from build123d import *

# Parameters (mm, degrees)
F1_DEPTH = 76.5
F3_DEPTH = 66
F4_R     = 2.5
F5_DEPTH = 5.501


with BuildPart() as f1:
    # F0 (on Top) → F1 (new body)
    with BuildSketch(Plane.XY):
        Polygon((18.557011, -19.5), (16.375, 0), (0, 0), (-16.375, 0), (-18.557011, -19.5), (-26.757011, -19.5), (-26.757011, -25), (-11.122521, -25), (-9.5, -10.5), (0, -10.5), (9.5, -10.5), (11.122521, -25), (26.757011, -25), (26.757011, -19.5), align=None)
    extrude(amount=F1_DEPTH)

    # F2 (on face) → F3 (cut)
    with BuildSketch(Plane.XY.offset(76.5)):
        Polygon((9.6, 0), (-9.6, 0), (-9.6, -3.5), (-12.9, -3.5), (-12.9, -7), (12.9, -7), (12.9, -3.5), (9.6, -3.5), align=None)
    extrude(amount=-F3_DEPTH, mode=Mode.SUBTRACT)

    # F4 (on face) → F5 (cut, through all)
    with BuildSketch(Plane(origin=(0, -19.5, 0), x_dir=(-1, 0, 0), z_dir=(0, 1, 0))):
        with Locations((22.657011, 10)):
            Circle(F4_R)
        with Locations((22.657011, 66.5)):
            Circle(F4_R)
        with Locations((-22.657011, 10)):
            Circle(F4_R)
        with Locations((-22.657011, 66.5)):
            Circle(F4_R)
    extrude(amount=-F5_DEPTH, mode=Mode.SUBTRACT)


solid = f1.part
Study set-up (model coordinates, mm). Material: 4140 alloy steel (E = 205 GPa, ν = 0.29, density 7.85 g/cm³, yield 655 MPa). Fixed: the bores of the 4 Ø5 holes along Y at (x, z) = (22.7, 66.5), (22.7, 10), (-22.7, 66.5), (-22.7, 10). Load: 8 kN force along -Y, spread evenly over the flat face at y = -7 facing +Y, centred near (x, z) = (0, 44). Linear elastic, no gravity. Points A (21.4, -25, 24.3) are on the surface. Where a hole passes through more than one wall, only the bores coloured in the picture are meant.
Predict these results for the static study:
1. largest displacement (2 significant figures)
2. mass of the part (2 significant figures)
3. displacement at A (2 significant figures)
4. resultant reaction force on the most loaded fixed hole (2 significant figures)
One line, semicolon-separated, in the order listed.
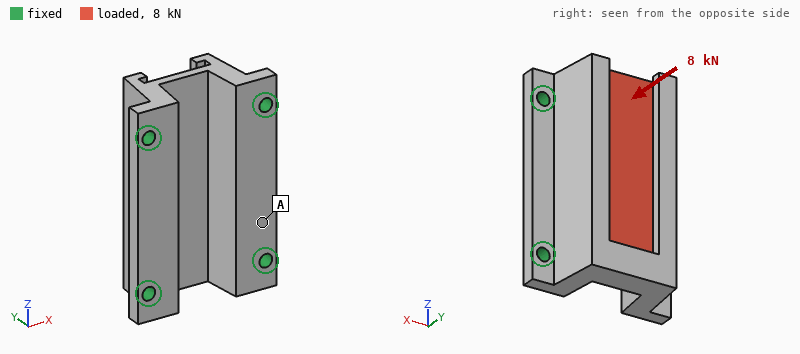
12 µm; 320 g; 4.0 µm; 3.1 kN
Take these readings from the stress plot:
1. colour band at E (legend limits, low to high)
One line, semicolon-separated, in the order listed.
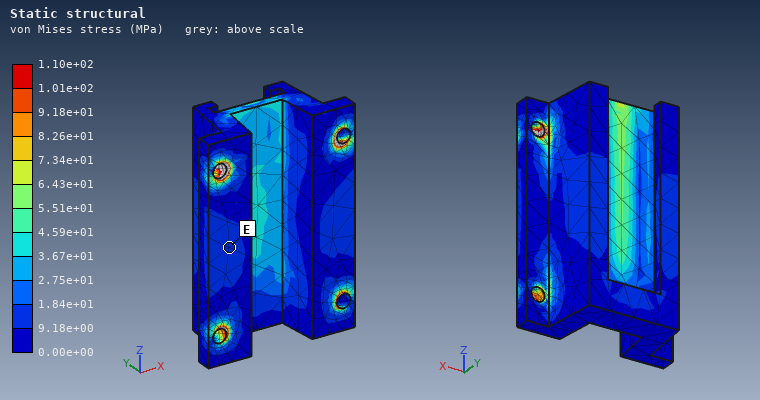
9.18e+00 to 1.84e+01 MPa
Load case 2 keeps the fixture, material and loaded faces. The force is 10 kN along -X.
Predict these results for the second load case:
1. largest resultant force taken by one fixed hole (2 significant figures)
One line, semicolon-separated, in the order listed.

3.2 kN
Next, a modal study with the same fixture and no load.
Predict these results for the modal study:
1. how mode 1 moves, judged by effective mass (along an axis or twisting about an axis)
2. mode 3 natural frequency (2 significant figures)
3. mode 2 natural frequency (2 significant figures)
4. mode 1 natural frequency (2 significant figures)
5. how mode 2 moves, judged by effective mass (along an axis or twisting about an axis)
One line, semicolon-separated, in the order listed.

along X; 12 kHz; 12 kHz; 8600 Hz; along Y
